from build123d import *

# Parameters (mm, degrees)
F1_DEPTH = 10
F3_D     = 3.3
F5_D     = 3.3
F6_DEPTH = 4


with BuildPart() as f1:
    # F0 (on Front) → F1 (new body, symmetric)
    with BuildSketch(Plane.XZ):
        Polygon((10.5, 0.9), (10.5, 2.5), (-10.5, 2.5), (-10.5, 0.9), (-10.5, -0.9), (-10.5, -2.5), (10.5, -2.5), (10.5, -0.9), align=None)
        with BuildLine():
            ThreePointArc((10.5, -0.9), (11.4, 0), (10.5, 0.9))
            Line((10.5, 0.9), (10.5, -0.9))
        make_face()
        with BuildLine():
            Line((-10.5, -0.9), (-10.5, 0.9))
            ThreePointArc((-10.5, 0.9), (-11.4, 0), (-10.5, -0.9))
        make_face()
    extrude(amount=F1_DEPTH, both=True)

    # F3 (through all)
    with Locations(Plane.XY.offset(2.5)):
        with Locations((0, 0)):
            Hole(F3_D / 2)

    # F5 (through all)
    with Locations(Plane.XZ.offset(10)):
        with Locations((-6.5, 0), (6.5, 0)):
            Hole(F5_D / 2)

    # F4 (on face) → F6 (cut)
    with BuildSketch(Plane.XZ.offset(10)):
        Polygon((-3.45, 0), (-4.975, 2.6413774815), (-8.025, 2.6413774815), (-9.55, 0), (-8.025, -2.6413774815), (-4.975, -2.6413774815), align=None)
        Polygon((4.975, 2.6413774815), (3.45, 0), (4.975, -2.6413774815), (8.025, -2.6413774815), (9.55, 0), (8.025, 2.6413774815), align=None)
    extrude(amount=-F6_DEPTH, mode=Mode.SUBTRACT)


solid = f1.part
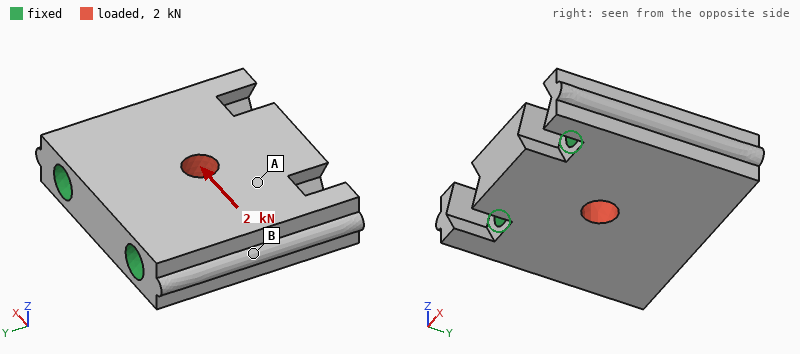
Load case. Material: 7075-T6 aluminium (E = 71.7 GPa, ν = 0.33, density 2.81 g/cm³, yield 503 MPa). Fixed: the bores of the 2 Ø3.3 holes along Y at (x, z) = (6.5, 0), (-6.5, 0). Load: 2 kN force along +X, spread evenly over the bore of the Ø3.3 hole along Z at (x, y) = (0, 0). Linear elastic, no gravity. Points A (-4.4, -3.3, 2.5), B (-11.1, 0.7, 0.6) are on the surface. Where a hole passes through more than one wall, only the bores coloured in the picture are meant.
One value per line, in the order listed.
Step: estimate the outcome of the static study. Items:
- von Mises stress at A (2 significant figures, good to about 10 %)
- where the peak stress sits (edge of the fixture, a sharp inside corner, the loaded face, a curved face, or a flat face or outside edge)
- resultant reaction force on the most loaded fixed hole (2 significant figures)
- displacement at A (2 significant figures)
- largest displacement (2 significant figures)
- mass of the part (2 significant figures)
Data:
14 MPa
the loaded face
1.0 kN
0.43 µm
1.9 µm
4.6 g
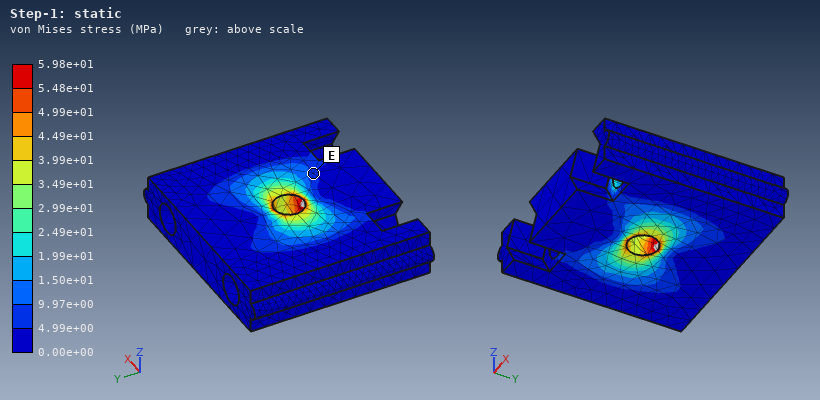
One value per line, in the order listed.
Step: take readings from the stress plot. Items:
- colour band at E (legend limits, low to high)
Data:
4.99e+00 to 9.97e+00 MPa
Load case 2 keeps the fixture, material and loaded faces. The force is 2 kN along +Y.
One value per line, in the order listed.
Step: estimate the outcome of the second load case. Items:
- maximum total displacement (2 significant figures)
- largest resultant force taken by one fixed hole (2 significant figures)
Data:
3.2 µm
1.0 kN
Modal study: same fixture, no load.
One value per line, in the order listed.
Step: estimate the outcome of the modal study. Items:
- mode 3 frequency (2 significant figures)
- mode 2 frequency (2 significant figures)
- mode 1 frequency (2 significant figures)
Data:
62 kHz
62 kHz
57 kHz
